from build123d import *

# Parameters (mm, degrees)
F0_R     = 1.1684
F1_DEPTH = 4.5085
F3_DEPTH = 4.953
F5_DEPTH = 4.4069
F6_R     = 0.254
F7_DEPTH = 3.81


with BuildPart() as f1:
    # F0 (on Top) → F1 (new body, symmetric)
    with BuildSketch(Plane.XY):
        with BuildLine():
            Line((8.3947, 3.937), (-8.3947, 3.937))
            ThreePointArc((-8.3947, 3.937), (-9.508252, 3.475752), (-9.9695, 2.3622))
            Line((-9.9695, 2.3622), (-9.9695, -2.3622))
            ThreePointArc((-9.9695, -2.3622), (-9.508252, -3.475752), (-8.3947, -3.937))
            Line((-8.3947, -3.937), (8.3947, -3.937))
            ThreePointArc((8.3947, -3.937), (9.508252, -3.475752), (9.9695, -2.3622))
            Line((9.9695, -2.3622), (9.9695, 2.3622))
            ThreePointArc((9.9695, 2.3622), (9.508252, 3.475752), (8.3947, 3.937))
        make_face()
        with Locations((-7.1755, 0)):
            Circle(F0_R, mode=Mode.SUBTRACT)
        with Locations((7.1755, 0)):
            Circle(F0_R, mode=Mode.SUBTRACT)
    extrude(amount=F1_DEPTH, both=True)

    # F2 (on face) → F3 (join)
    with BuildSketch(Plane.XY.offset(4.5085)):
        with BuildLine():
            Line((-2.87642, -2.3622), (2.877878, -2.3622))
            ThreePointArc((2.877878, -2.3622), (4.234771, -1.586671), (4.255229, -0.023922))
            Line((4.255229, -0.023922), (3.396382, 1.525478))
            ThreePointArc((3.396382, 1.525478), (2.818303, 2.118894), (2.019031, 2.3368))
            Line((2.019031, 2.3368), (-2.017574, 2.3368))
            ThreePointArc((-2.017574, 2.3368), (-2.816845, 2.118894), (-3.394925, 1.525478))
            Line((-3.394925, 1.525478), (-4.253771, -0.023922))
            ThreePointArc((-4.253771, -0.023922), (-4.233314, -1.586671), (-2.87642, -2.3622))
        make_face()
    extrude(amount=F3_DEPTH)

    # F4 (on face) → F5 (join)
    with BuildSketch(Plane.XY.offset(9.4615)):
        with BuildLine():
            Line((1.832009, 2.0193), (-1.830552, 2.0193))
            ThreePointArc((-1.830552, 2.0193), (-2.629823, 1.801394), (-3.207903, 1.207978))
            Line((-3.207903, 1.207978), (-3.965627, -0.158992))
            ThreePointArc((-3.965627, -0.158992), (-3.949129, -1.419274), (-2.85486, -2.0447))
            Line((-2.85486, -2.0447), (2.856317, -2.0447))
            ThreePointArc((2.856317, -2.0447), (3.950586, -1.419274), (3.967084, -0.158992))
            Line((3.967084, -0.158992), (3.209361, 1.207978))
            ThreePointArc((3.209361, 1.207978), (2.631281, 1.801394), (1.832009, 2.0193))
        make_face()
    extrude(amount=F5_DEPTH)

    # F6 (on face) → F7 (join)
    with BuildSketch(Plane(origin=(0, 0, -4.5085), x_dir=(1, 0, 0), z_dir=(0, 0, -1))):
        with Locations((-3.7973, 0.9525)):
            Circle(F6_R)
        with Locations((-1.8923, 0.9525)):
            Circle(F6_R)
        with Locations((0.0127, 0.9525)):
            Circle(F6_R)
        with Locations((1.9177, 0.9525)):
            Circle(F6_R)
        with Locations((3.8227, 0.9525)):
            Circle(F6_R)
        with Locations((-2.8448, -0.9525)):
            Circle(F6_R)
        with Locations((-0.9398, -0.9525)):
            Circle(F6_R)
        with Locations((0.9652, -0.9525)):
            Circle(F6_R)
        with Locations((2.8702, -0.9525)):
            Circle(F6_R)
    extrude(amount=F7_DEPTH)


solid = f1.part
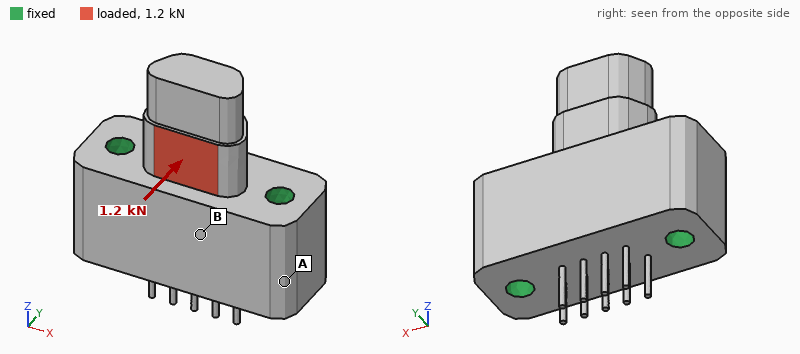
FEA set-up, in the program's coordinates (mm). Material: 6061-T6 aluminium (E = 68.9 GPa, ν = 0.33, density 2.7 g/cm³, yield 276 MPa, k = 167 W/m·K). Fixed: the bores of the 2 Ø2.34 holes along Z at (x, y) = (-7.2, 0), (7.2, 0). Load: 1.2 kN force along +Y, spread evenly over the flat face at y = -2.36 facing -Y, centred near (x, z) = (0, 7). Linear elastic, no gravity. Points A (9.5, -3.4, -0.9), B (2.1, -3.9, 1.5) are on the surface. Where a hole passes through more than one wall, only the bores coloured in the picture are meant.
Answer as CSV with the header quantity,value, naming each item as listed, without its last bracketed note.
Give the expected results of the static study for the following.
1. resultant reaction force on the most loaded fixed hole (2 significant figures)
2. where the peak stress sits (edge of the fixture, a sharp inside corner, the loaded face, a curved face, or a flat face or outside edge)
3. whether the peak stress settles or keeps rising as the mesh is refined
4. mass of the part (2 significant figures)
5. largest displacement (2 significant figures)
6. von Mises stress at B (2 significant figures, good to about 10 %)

quantity,value
resultant reaction force on the most loaded fixed hole,600 N
where the peak stress sits,edge of the fixture
whether the peak stress settles or keeps rising as the mesh is refined,keeps rising
mass of the part,4.4 g
largest displacement,42 µm
von Mises stress at B,55 MPa
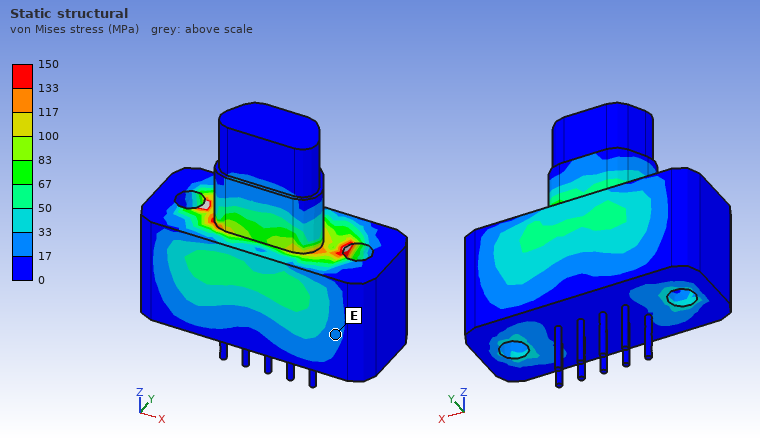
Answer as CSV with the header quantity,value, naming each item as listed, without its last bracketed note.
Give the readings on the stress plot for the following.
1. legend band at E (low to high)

quantity,value
legend band at E,17 to 33 MPa
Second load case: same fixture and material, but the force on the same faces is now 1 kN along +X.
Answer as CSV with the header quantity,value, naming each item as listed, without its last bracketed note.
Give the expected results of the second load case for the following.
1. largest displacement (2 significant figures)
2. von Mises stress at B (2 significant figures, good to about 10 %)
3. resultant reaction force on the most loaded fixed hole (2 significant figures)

quantity,value
largest displacement,15 µm
von Mises stress at B,7.9 MPa
resultant reaction force on the most loaded fixed hole,670 N
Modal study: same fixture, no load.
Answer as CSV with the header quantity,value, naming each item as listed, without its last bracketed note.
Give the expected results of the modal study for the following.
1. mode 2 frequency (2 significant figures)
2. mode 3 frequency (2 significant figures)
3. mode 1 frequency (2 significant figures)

quantity,value
mode 2 frequency,23 kHz
mode 3 frequency,23 kHz
mode 1 frequency,23 kHz
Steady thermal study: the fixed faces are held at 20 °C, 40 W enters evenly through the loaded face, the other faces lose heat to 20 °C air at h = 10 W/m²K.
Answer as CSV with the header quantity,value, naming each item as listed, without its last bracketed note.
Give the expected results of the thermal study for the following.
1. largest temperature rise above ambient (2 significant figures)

quantity,value
largest temperature rise above ambient,44 K
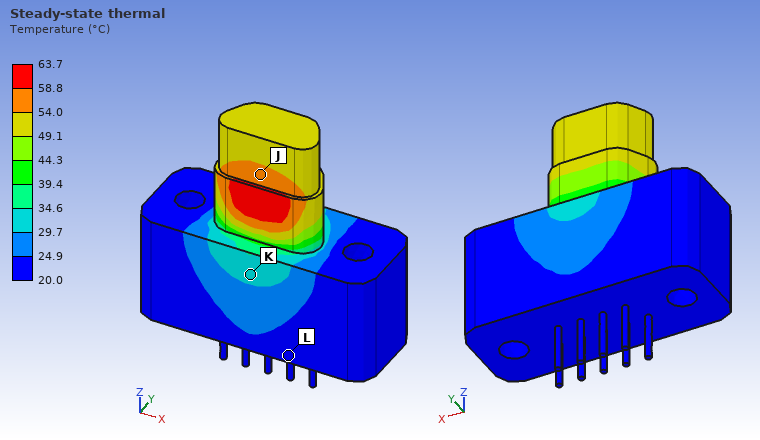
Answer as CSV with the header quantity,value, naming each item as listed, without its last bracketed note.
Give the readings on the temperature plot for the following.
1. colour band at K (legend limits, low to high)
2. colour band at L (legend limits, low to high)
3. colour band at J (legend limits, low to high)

quantity,value
colour band at K,29.7 to 34.6 °C
colour band at L,20.0 to 24.9 °C
colour band at J,54.0 to 58.8 °C
